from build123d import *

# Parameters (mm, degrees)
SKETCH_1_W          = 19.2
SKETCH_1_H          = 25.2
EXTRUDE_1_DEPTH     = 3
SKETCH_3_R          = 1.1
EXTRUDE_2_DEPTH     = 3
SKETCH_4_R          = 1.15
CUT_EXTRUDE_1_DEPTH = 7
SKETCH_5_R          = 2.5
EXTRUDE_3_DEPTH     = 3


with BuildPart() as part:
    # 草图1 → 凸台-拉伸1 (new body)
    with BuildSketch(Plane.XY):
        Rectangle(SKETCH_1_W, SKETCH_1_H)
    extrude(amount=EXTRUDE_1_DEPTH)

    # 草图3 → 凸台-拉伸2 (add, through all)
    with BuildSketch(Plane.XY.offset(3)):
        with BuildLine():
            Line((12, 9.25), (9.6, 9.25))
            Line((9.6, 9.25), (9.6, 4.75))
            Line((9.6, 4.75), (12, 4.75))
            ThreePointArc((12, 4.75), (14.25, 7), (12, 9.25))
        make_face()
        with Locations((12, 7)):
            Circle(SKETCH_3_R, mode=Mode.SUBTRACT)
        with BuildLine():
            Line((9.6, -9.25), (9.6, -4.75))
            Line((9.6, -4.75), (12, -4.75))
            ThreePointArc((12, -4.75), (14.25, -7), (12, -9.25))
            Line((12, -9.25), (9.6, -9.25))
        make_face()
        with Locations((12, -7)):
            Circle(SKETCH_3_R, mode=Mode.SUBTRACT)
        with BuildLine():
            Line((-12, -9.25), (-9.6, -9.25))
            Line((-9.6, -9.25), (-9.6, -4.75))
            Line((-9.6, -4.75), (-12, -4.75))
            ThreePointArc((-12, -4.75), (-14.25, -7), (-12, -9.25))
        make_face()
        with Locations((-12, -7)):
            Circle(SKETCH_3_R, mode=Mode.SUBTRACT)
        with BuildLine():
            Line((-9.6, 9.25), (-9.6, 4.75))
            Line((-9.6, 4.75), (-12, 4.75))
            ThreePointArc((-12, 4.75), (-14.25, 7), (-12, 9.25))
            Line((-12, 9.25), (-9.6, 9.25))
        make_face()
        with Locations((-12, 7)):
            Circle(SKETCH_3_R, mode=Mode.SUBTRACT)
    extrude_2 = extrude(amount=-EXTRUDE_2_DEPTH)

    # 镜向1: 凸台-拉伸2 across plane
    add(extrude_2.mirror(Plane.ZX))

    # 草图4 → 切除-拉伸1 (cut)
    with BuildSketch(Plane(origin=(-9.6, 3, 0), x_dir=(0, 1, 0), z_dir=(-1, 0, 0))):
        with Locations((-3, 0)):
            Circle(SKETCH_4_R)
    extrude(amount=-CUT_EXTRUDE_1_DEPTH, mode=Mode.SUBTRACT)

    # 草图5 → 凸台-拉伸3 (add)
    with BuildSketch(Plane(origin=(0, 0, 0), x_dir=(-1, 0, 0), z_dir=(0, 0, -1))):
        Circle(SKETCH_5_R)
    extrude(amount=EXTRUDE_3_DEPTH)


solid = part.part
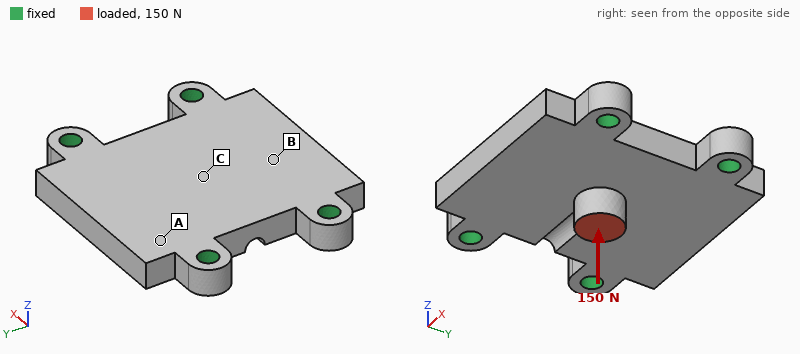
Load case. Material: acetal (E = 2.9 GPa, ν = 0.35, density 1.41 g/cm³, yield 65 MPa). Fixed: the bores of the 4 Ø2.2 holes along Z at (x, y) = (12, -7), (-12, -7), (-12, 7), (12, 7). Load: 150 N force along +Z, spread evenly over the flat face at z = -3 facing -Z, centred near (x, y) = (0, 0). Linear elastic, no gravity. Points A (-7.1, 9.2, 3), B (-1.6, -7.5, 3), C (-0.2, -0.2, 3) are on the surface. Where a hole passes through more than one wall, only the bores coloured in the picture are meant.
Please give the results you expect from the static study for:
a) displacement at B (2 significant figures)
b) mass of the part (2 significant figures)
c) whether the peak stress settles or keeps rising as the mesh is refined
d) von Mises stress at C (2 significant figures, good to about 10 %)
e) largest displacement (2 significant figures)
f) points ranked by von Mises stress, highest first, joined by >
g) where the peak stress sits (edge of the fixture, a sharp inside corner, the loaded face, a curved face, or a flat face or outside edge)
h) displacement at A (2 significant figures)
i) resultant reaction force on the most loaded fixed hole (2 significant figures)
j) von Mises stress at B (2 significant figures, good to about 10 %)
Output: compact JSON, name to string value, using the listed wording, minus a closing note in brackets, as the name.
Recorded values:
{"displacement at B": "0.078 mm", "mass of the part": "2.4 g", "whether the peak stress settles or keeps rising as the mesh is refined": "keeps rising", "von Mises stress at C": "16 MPa", "largest displacement": "0.14 mm", "points ranked by von Mises stress, highest first, joined by >": "C > B > A", "where the peak stress sits": "a sharp inside corner", "displacement at A": "0.029 mm", "resultant reaction force on the most loaded fixed hole": "38 N", "von Mises stress at B": "8.2 MPa"}
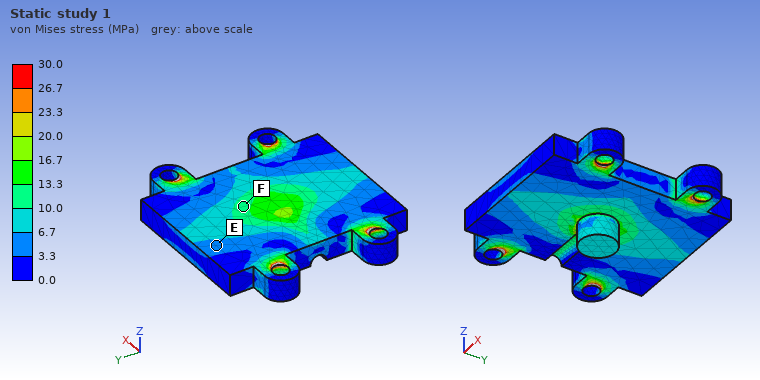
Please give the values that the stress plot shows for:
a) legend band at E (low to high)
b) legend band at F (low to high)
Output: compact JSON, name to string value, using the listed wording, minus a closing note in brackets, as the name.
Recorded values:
{"legend band at E": "3.3 to 6.7 MPa", "legend band at F": "10.0 to 13.3 MPa"}
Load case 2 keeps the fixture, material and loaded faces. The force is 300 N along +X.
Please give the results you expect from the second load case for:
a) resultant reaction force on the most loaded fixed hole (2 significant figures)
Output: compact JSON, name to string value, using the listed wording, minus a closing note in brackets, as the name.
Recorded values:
{"resultant reaction force on the most loaded fixed hole": "90 N"}
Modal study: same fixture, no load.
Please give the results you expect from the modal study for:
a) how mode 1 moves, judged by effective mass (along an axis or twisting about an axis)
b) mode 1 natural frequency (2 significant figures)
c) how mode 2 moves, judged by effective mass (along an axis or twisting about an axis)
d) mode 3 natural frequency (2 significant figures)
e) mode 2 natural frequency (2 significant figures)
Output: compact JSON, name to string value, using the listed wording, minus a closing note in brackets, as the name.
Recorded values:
{"how mode 1 moves, judged by effective mass": "along Z", "mode 1 natural frequency": "5700 Hz", "how mode 2 moves, judged by effective mass": "twisting about X", "mode 3 natural frequency": "8900 Hz", "mode 2 natural frequency": "6400 Hz"}
